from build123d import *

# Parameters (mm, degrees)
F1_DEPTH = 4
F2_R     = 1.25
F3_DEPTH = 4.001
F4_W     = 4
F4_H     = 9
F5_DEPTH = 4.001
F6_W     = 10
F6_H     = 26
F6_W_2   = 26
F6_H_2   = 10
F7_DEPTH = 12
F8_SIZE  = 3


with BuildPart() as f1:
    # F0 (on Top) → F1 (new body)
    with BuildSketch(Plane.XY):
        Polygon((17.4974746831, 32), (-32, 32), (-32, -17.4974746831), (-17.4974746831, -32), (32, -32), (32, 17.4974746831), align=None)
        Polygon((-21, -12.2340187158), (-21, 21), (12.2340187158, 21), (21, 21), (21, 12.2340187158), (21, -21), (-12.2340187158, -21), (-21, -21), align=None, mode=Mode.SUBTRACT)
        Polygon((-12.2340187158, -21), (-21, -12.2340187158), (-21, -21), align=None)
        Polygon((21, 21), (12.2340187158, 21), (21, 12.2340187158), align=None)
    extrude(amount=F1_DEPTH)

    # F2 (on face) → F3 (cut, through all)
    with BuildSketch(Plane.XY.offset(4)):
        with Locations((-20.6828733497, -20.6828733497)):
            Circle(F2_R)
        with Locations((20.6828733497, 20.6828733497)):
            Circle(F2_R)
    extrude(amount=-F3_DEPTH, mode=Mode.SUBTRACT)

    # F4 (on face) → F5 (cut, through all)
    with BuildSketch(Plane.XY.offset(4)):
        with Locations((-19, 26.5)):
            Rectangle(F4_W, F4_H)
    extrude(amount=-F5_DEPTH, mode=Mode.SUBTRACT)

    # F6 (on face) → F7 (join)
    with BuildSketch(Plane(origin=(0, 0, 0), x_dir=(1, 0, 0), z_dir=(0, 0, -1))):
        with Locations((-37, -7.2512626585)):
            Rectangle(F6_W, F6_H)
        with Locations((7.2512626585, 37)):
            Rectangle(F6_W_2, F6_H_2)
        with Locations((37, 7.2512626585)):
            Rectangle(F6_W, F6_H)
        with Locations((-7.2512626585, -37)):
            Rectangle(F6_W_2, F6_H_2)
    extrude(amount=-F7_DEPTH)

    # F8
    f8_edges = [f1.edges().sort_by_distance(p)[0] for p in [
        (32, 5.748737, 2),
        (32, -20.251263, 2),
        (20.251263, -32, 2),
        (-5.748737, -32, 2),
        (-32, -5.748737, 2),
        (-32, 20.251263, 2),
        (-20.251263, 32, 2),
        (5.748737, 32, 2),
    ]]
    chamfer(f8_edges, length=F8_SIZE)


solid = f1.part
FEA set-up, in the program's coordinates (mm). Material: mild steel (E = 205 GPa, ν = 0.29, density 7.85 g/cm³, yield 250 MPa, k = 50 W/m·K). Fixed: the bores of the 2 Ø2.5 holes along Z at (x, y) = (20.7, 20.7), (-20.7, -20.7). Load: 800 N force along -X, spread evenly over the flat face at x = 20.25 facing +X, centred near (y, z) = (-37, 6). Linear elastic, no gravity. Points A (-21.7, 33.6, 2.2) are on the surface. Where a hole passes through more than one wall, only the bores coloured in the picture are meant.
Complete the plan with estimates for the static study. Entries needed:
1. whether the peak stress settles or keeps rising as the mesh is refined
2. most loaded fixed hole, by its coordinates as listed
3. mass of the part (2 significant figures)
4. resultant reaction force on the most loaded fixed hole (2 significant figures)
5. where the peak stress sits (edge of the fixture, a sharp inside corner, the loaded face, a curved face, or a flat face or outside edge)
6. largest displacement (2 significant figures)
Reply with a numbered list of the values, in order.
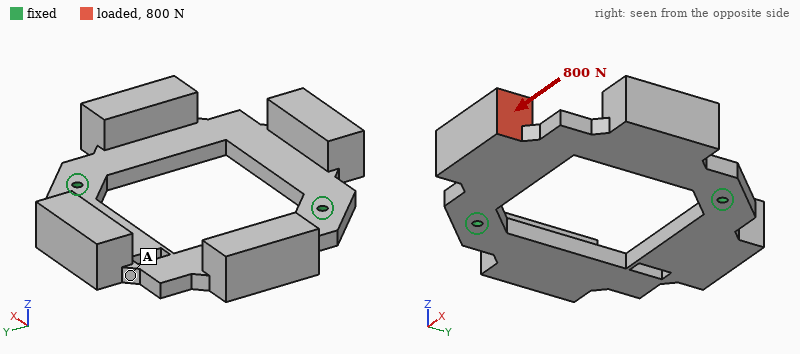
1. keeps rising
2. (-20.7, -20.7)
3. 170 g
4. 860 N
5. edge of the fixture
6. 94 µm
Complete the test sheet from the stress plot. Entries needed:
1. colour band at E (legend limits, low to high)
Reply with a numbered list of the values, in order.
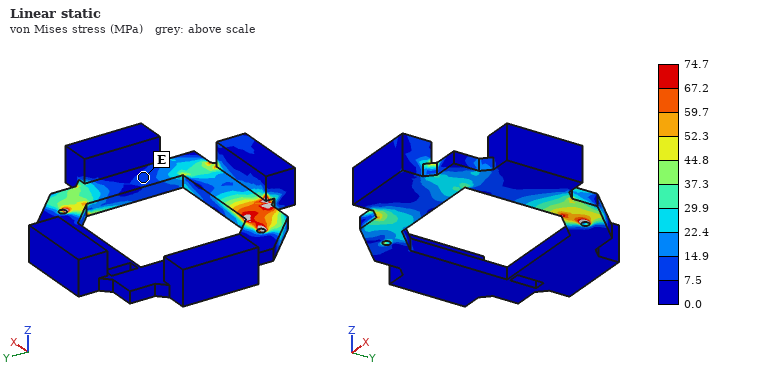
1. 7.5 to 14.9 MPa
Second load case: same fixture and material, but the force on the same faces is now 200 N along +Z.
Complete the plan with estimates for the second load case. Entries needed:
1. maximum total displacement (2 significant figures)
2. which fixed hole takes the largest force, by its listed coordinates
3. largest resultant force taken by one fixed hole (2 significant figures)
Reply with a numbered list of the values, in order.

1. 0.23 mm
2. (-20.7, -20.7)
3. 130 N
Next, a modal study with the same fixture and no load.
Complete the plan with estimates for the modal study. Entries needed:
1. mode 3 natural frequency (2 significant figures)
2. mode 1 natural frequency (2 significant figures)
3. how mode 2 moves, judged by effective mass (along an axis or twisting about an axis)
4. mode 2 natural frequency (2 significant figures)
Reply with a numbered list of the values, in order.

1. 2300 Hz
2. 860 Hz
3. along Z
4. 920 Hz
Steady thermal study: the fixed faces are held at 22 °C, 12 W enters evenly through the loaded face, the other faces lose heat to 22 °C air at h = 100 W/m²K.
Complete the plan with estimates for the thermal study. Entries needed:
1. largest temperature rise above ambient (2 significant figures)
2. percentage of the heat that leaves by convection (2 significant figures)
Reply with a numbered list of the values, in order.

1. 53 K
2. 75 %
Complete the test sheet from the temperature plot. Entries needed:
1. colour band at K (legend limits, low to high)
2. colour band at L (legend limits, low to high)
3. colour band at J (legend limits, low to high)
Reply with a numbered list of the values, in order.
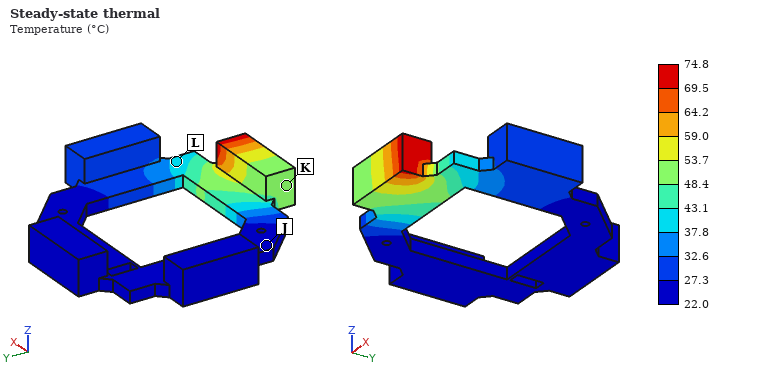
1. 48.4 to 53.7 °C
2. 37.8 to 43.1 °C
3. 22.0 to 27.3 °C
